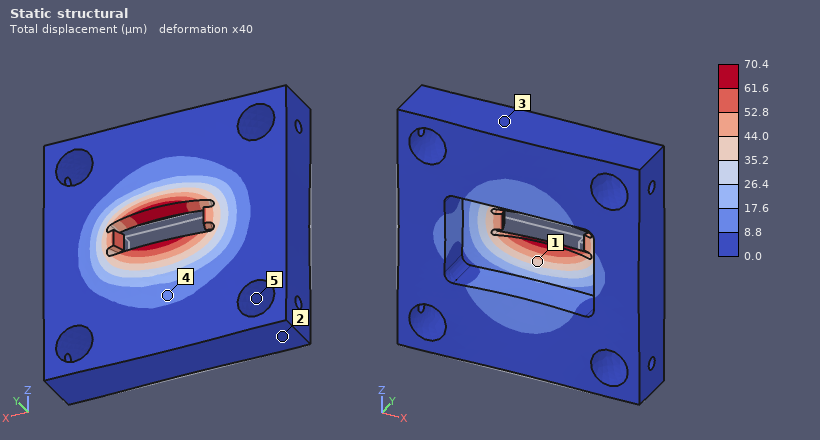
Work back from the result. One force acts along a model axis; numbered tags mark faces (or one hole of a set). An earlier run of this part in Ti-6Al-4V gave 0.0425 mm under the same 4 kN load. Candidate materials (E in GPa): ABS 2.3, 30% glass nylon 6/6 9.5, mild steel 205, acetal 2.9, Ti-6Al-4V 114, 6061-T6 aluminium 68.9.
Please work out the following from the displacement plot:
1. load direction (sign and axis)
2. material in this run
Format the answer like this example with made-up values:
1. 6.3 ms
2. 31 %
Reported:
1. +Y
2. 6061-T6 aluminium
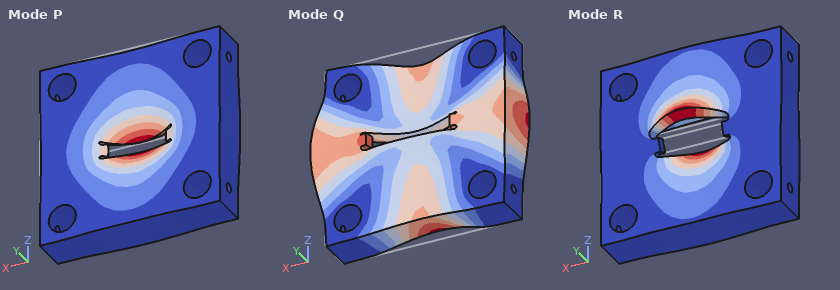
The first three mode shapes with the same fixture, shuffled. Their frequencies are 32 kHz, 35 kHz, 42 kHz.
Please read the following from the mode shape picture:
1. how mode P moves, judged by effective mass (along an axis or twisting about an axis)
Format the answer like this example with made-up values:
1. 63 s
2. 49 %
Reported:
1. along Y
